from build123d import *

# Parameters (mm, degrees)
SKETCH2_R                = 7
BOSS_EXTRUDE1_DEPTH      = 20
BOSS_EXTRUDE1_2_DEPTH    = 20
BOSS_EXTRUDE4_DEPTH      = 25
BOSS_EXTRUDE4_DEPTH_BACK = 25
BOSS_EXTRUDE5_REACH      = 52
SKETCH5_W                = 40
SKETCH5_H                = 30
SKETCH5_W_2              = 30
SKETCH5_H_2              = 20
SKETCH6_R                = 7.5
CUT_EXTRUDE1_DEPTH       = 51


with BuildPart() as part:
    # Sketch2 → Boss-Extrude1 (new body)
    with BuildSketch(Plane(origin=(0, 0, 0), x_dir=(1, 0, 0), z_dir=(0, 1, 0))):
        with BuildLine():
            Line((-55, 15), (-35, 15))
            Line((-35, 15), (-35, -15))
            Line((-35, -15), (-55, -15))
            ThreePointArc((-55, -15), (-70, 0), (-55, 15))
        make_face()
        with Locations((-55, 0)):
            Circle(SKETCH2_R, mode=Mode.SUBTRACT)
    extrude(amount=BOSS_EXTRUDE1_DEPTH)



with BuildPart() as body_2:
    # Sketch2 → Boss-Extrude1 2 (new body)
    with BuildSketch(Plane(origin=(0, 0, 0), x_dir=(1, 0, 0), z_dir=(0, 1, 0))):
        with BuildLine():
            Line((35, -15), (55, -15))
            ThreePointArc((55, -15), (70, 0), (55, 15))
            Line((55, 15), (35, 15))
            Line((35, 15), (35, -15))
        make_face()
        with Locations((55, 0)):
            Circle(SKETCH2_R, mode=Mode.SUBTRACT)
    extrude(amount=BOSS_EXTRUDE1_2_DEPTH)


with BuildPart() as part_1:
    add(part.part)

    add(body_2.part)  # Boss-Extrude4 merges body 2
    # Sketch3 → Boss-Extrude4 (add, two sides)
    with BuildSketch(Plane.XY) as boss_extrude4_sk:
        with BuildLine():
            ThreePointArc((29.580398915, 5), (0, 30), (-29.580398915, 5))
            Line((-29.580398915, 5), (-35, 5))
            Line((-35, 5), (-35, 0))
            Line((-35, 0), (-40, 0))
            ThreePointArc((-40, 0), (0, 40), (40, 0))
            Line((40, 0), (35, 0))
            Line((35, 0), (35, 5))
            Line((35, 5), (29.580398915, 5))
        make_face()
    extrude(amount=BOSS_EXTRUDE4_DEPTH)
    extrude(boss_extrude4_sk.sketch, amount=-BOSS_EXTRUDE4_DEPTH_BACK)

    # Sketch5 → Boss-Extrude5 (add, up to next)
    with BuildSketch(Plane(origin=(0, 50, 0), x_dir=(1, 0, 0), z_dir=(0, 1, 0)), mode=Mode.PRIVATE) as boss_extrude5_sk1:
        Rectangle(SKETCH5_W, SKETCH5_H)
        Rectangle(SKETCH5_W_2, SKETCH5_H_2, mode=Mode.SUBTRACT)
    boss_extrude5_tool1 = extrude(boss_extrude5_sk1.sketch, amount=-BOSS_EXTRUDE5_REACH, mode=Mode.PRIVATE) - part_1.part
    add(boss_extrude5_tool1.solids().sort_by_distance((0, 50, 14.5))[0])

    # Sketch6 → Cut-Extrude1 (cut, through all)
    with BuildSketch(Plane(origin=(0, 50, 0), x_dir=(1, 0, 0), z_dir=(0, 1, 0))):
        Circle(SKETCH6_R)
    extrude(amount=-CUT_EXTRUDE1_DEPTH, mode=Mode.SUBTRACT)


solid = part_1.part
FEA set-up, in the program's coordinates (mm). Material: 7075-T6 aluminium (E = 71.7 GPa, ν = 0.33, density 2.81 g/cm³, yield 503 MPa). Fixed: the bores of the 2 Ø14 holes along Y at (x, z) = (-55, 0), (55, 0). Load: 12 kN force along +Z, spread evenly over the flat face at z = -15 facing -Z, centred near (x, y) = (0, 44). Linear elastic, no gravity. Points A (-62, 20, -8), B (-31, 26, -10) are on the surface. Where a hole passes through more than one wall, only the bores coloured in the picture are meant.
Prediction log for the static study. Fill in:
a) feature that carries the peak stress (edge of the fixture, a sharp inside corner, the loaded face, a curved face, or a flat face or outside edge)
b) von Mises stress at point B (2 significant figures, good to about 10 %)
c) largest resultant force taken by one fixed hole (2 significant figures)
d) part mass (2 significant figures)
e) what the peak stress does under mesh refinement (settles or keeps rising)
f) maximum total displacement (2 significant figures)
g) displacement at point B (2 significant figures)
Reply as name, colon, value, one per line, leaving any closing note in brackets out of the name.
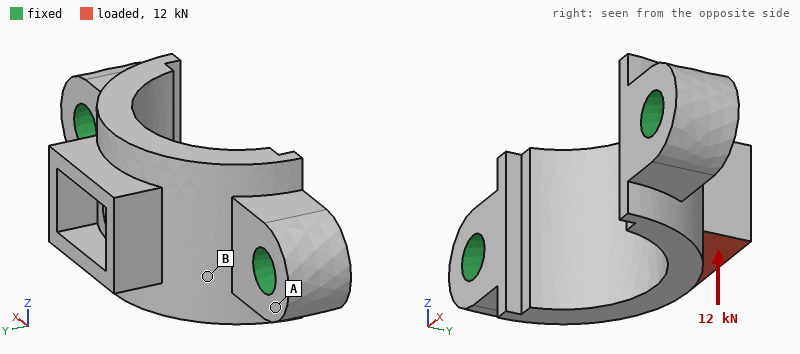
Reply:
feature that carries the peak stress: edge of the fixture
von Mises stress at point B: 57 MPa
largest resultant force taken by one fixed hole: 6.0 kN
part mass: 240 g
what the peak stress does under mesh refinement: keeps rising
maximum total displacement: 0.30 mm
displacement at point B: 0.084 mm
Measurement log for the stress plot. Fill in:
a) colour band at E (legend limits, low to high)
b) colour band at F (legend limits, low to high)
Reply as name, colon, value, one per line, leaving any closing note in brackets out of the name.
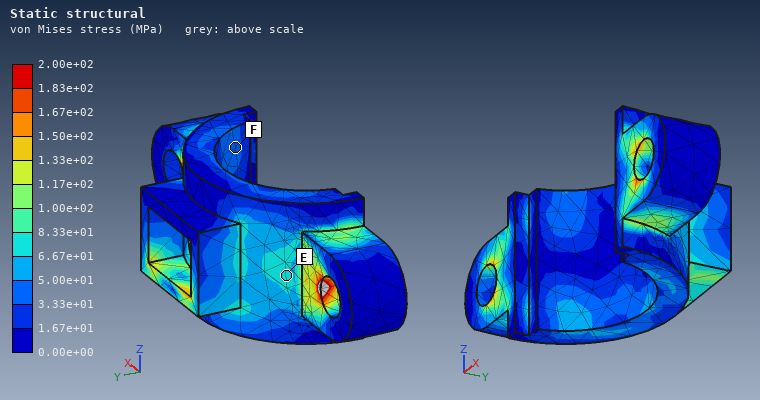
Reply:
colour band at E: 6.67e+01 to 8.33e+01 MPa
colour band at F: 3.33e+01 to 5.00e+01 MPa
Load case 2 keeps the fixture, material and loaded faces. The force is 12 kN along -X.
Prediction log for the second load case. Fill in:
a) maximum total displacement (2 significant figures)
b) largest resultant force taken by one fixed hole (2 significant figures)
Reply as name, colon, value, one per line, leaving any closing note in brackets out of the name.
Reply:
maximum total displacement: 59 µm
largest resultant force taken by one fixed hole: 7.9 kN
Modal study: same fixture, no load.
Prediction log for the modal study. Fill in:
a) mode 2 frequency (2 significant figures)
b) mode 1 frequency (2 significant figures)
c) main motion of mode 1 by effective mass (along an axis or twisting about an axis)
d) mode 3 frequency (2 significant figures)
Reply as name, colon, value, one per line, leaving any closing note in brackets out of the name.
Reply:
mode 2 frequency: 10000 Hz
mode 1 frequency: 4700 Hz
main motion of mode 1 by effective mass: along Z
mode 3 frequency: 10 kHz
